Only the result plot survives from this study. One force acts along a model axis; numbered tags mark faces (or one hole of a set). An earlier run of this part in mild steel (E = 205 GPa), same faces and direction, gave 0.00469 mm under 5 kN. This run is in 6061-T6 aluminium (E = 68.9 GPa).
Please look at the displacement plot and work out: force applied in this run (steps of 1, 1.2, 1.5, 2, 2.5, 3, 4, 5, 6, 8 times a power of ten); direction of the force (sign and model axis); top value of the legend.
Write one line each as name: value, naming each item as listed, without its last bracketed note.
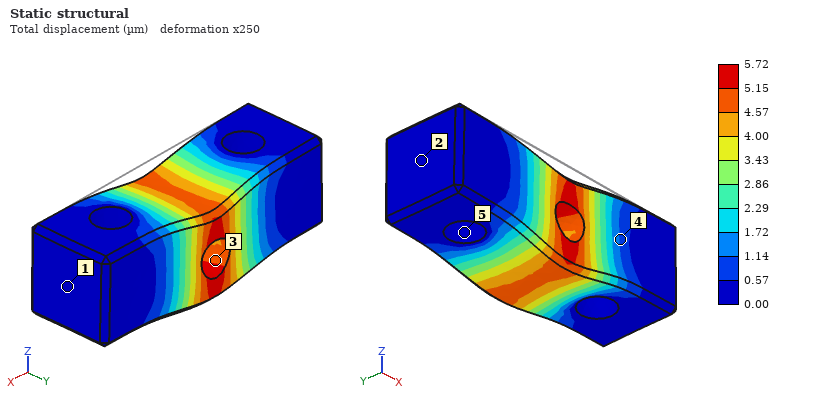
force applied in this run: 2 kN
direction of the force: -Z
top value of the legend: 5.72 µm
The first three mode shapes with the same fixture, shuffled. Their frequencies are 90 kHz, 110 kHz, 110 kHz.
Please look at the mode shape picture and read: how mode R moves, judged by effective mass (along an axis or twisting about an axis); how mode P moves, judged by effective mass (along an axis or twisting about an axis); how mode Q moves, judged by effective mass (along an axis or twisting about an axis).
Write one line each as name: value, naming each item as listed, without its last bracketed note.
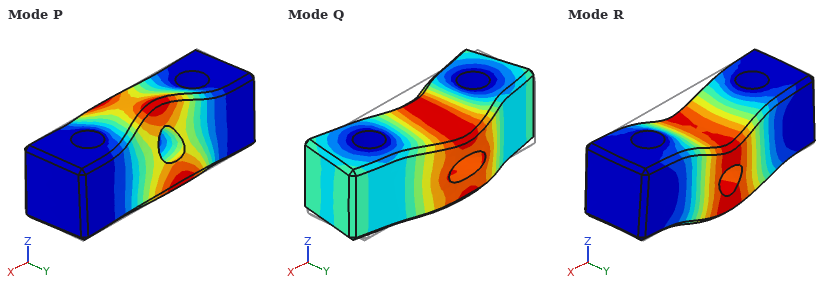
how mode R moves, judged by effective mass: along Z
how mode P moves, judged by effective mass: twisting about X
how mode Q moves, judged by effective mass: along Y
